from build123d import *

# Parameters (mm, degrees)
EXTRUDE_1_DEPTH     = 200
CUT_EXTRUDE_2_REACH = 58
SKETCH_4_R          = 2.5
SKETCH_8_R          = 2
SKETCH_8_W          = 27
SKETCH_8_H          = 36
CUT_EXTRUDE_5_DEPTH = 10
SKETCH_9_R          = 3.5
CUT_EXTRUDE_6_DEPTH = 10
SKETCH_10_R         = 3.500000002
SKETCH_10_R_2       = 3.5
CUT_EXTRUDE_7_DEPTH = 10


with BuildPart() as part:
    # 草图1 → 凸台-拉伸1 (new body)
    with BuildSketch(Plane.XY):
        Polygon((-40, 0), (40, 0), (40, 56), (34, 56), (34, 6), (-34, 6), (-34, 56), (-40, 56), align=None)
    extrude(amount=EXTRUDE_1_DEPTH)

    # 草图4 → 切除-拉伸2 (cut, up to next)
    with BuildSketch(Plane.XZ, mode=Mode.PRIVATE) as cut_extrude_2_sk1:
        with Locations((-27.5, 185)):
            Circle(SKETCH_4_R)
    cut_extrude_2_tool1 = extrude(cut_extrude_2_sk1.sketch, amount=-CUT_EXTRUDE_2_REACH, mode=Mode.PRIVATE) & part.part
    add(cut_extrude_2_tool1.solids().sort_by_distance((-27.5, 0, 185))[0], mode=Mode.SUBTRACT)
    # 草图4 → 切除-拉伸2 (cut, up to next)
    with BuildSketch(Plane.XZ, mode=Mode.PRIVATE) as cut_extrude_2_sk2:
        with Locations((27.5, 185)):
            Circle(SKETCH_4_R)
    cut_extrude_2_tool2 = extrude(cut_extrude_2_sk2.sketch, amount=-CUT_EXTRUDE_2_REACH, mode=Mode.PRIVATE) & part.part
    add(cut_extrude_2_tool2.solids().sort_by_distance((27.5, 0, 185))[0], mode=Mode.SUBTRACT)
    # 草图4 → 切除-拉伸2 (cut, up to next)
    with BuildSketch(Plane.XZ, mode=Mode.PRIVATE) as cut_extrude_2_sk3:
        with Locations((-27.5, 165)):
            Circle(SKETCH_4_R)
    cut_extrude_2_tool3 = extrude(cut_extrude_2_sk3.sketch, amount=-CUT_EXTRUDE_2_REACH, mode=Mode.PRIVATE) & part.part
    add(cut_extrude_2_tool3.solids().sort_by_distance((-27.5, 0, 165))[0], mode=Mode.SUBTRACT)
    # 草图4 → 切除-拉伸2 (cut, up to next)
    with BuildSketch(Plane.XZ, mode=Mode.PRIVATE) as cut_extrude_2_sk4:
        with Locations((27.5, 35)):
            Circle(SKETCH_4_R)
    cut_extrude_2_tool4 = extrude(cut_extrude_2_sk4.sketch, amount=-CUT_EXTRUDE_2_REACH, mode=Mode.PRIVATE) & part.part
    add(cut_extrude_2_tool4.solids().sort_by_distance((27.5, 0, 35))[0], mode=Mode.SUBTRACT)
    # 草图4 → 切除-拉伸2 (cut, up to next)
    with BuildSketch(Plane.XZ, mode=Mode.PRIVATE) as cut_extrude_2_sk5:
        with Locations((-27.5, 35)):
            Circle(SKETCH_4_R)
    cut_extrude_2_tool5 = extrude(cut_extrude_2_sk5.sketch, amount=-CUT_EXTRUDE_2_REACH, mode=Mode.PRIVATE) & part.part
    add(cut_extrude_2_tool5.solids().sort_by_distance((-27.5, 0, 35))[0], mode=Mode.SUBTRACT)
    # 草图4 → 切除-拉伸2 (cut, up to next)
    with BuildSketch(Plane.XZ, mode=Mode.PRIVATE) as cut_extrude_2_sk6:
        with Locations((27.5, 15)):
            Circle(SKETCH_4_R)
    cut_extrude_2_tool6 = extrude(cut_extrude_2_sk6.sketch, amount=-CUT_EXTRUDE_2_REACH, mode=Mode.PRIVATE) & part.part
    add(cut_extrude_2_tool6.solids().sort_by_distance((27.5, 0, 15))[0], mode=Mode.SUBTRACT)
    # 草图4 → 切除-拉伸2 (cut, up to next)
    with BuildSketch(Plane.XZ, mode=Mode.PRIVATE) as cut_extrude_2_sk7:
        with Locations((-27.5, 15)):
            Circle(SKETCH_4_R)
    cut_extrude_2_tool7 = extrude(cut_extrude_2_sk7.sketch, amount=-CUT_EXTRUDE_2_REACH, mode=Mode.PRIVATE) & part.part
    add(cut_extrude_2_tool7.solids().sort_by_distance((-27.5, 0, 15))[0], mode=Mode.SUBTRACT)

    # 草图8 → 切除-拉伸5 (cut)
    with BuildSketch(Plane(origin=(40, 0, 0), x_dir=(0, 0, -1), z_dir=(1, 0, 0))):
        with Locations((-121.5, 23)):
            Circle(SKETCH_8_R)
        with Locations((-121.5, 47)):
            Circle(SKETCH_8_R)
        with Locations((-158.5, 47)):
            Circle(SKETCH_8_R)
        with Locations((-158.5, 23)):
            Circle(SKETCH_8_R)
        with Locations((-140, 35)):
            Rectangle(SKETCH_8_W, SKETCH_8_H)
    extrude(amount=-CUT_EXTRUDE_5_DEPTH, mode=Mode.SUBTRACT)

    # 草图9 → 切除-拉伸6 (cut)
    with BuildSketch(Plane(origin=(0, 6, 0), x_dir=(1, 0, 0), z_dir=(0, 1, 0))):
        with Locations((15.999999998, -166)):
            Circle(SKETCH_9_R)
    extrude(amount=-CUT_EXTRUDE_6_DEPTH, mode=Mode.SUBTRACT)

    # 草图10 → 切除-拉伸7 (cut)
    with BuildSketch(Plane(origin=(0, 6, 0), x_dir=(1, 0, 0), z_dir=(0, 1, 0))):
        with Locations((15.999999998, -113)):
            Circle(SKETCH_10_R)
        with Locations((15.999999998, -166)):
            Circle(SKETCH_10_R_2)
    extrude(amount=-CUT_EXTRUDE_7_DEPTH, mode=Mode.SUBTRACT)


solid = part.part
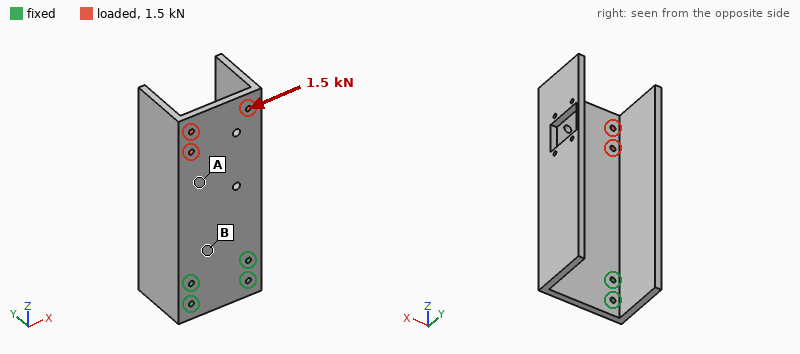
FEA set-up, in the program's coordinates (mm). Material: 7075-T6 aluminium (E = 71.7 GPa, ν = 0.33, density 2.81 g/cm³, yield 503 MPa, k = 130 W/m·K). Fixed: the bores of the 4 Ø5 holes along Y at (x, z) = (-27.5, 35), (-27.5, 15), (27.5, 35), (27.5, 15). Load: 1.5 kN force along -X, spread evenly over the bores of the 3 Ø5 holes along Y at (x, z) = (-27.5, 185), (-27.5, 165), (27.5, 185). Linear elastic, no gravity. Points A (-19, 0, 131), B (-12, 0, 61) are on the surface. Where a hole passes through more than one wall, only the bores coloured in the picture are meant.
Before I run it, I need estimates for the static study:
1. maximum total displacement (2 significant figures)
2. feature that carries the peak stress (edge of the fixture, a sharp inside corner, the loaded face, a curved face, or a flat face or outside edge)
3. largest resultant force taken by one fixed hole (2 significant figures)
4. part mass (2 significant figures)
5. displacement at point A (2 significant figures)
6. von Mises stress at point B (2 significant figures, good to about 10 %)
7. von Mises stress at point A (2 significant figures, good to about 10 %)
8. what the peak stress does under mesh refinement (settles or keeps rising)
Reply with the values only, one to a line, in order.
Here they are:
0.14 mm
edge of the fixture
2.7 kN
590 g
0.046 mm
9.7 MPa
4.8 MPa
keeps rising
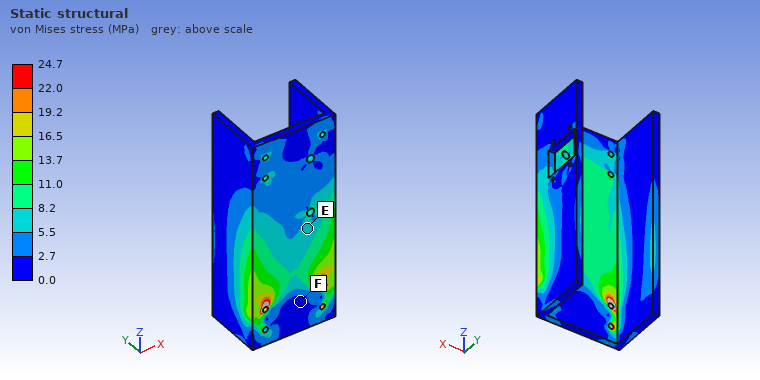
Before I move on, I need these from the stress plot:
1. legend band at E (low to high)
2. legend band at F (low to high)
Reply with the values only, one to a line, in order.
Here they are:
5.5 to 8.2 MPa
0.0 to 2.7 MPa
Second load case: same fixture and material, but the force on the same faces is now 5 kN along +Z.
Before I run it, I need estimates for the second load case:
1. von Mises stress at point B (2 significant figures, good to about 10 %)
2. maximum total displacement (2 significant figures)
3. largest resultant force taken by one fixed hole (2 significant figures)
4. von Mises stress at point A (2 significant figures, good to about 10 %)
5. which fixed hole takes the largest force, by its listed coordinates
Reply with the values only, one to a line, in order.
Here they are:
10 MPa
67 µm
2.3 kN
12 MPa
(-27.5, 35)
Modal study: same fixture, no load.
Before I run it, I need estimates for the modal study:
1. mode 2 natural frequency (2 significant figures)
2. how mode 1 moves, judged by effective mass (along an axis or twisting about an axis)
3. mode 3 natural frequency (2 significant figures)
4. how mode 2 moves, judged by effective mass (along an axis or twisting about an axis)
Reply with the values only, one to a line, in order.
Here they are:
590 Hz
along Y
1000 Hz
along X
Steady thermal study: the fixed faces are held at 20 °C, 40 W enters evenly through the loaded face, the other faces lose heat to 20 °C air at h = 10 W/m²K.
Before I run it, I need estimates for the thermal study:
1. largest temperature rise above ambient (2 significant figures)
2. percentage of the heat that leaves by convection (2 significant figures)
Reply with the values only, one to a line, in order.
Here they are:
46 K
34 %
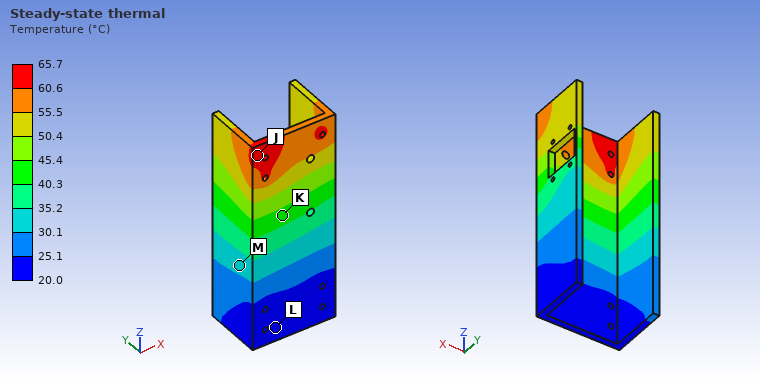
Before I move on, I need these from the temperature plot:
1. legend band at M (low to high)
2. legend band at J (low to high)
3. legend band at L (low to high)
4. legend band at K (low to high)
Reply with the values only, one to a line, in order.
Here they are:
30.1 to 35.2 °C
60.6 to 65.7 °C
20.0 to 25.1 °C
40.3 to 45.4 °C
